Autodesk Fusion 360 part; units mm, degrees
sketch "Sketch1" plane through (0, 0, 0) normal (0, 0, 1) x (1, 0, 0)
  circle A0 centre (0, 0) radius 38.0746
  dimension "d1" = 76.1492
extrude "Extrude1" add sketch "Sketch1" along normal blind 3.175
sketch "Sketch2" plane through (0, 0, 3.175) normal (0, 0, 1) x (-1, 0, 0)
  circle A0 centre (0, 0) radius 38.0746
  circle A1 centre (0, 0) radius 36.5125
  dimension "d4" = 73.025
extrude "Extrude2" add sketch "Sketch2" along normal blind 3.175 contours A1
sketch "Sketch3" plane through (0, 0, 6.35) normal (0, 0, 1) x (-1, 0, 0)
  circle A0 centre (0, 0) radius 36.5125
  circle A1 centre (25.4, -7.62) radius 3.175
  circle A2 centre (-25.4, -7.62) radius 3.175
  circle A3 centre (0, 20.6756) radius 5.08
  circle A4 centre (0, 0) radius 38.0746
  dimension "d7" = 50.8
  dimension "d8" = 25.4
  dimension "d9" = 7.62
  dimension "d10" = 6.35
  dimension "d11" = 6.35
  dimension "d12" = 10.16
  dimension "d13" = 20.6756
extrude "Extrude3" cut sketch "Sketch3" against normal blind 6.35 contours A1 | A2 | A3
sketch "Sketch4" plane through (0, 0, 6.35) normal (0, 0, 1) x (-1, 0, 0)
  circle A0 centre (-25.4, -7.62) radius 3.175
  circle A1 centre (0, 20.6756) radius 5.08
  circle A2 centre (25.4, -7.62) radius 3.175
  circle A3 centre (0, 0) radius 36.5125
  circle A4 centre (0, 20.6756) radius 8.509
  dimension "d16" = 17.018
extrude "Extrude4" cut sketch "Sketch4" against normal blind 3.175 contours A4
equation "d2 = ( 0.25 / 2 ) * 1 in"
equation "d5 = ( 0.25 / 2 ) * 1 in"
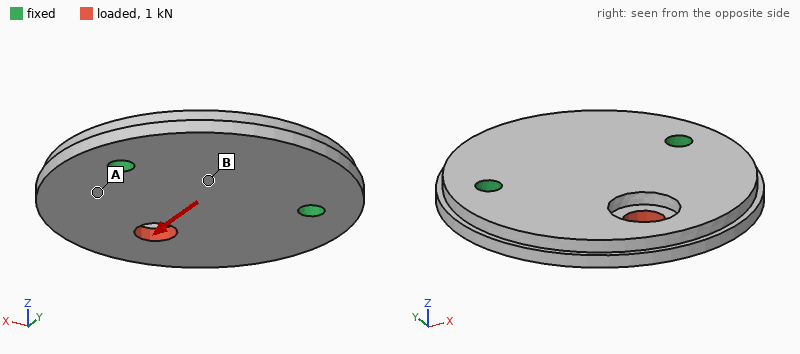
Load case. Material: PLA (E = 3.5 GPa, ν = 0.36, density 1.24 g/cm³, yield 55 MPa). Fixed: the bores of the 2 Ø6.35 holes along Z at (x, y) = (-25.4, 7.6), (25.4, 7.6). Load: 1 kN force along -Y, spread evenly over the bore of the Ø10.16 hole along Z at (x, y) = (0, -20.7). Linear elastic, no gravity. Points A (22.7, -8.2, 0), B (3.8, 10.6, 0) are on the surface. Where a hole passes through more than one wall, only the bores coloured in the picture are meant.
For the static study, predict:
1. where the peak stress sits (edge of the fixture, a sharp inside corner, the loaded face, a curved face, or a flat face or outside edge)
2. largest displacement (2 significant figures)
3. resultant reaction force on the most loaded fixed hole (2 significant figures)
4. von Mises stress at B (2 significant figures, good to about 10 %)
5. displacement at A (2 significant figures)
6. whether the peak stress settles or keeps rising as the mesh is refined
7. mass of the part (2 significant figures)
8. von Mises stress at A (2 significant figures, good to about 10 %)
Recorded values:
a sharp inside corner
0.33 mm
520 N
2.5 MPa
0.050 mm
keeps rising
33 g
5.5 MPa
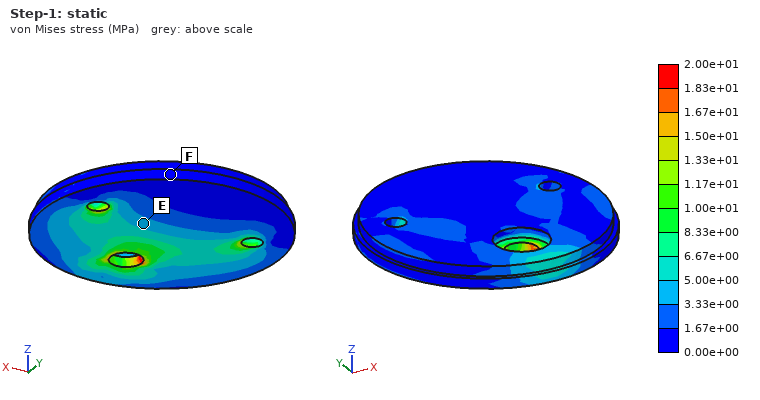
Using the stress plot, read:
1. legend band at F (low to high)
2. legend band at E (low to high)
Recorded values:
0.00e+00 to 1.67e+00 MPa
3.33e+00 to 5.00e+00 MPa
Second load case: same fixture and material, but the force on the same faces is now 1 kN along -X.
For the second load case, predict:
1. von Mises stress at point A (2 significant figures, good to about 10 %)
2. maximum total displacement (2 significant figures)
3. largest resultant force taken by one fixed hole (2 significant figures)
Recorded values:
4.5 MPa
0.12 mm
720 N
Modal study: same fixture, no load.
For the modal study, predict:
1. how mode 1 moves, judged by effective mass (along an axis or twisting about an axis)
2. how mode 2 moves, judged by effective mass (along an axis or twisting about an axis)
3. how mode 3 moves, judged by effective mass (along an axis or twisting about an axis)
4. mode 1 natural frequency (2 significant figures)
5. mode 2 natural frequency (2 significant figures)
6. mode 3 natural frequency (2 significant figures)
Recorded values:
along Z
along Z
twisting about Y
1000 Hz
2000 Hz
2200 Hz
